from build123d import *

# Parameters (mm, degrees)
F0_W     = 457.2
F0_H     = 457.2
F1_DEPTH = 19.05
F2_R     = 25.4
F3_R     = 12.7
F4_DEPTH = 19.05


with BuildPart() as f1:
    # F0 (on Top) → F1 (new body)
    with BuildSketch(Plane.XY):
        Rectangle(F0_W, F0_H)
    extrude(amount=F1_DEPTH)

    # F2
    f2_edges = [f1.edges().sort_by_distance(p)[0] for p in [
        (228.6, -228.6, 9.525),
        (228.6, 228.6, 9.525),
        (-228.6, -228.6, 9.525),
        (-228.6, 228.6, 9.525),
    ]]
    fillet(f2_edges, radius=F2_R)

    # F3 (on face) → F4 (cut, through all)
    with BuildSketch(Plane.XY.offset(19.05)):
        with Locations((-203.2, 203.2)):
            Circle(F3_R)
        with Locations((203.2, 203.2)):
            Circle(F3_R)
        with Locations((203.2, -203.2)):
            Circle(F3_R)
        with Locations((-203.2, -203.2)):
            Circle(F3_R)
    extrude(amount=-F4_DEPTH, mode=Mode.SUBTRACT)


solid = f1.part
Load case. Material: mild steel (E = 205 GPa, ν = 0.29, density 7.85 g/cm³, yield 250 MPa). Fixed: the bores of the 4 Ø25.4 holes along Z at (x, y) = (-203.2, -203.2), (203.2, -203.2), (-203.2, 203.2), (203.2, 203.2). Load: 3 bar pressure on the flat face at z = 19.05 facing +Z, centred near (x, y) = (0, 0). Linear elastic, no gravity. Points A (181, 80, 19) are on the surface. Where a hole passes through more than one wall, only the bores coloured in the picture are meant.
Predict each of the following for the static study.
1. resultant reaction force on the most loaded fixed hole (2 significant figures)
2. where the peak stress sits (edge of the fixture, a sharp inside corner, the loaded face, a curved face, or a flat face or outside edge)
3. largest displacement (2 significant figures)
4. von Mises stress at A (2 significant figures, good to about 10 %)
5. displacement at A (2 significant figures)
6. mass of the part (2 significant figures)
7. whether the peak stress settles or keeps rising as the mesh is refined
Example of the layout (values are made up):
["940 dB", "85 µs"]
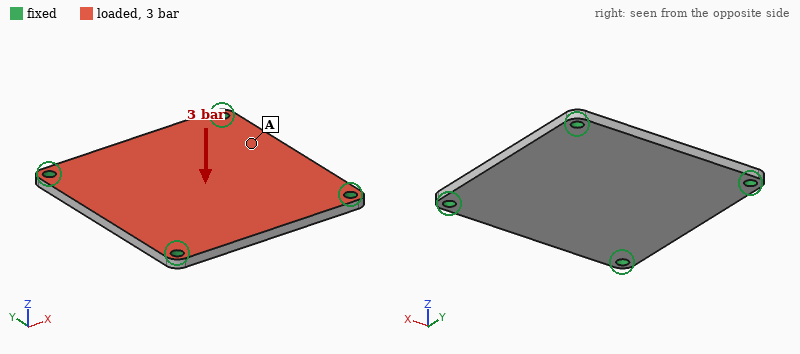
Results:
["15 kN", "edge of the fixture", "0.50 mm", "30 MPa", "0.23 mm", "31 kg", "keeps rising"]
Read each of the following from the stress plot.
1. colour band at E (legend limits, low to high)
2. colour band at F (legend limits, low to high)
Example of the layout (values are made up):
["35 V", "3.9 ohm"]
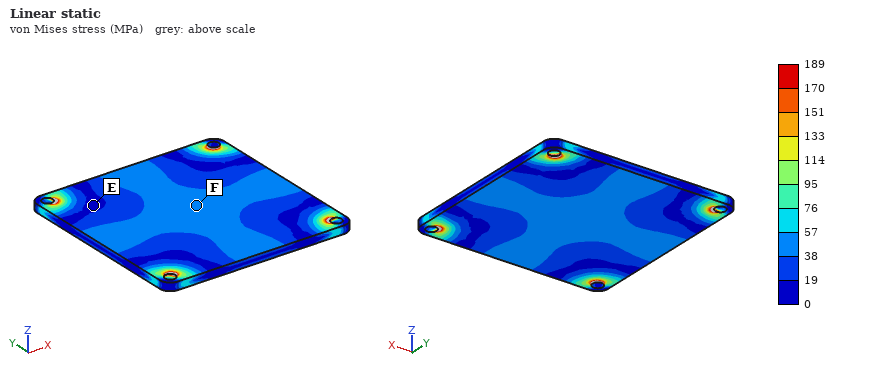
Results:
["0 to 19 MPa", "38 to 57 MPa"]
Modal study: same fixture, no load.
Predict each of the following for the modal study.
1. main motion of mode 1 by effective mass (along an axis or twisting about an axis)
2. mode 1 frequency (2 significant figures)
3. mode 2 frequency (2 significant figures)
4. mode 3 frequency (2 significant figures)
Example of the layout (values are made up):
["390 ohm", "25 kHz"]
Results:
["along Z", "380 Hz", "680 Hz", "680 Hz"]
